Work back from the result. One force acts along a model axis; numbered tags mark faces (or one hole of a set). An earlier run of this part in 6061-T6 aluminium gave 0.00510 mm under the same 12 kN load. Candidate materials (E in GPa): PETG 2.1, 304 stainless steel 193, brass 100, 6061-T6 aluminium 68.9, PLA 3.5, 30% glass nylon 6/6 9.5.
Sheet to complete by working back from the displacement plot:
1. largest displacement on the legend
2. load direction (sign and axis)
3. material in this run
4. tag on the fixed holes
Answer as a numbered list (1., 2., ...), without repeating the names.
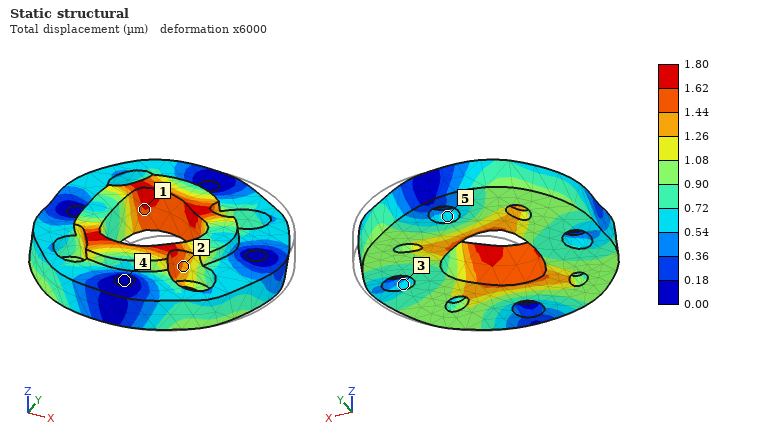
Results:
1. 1.80 µm
2. -X
3. 304 stainless steel
4. 4
